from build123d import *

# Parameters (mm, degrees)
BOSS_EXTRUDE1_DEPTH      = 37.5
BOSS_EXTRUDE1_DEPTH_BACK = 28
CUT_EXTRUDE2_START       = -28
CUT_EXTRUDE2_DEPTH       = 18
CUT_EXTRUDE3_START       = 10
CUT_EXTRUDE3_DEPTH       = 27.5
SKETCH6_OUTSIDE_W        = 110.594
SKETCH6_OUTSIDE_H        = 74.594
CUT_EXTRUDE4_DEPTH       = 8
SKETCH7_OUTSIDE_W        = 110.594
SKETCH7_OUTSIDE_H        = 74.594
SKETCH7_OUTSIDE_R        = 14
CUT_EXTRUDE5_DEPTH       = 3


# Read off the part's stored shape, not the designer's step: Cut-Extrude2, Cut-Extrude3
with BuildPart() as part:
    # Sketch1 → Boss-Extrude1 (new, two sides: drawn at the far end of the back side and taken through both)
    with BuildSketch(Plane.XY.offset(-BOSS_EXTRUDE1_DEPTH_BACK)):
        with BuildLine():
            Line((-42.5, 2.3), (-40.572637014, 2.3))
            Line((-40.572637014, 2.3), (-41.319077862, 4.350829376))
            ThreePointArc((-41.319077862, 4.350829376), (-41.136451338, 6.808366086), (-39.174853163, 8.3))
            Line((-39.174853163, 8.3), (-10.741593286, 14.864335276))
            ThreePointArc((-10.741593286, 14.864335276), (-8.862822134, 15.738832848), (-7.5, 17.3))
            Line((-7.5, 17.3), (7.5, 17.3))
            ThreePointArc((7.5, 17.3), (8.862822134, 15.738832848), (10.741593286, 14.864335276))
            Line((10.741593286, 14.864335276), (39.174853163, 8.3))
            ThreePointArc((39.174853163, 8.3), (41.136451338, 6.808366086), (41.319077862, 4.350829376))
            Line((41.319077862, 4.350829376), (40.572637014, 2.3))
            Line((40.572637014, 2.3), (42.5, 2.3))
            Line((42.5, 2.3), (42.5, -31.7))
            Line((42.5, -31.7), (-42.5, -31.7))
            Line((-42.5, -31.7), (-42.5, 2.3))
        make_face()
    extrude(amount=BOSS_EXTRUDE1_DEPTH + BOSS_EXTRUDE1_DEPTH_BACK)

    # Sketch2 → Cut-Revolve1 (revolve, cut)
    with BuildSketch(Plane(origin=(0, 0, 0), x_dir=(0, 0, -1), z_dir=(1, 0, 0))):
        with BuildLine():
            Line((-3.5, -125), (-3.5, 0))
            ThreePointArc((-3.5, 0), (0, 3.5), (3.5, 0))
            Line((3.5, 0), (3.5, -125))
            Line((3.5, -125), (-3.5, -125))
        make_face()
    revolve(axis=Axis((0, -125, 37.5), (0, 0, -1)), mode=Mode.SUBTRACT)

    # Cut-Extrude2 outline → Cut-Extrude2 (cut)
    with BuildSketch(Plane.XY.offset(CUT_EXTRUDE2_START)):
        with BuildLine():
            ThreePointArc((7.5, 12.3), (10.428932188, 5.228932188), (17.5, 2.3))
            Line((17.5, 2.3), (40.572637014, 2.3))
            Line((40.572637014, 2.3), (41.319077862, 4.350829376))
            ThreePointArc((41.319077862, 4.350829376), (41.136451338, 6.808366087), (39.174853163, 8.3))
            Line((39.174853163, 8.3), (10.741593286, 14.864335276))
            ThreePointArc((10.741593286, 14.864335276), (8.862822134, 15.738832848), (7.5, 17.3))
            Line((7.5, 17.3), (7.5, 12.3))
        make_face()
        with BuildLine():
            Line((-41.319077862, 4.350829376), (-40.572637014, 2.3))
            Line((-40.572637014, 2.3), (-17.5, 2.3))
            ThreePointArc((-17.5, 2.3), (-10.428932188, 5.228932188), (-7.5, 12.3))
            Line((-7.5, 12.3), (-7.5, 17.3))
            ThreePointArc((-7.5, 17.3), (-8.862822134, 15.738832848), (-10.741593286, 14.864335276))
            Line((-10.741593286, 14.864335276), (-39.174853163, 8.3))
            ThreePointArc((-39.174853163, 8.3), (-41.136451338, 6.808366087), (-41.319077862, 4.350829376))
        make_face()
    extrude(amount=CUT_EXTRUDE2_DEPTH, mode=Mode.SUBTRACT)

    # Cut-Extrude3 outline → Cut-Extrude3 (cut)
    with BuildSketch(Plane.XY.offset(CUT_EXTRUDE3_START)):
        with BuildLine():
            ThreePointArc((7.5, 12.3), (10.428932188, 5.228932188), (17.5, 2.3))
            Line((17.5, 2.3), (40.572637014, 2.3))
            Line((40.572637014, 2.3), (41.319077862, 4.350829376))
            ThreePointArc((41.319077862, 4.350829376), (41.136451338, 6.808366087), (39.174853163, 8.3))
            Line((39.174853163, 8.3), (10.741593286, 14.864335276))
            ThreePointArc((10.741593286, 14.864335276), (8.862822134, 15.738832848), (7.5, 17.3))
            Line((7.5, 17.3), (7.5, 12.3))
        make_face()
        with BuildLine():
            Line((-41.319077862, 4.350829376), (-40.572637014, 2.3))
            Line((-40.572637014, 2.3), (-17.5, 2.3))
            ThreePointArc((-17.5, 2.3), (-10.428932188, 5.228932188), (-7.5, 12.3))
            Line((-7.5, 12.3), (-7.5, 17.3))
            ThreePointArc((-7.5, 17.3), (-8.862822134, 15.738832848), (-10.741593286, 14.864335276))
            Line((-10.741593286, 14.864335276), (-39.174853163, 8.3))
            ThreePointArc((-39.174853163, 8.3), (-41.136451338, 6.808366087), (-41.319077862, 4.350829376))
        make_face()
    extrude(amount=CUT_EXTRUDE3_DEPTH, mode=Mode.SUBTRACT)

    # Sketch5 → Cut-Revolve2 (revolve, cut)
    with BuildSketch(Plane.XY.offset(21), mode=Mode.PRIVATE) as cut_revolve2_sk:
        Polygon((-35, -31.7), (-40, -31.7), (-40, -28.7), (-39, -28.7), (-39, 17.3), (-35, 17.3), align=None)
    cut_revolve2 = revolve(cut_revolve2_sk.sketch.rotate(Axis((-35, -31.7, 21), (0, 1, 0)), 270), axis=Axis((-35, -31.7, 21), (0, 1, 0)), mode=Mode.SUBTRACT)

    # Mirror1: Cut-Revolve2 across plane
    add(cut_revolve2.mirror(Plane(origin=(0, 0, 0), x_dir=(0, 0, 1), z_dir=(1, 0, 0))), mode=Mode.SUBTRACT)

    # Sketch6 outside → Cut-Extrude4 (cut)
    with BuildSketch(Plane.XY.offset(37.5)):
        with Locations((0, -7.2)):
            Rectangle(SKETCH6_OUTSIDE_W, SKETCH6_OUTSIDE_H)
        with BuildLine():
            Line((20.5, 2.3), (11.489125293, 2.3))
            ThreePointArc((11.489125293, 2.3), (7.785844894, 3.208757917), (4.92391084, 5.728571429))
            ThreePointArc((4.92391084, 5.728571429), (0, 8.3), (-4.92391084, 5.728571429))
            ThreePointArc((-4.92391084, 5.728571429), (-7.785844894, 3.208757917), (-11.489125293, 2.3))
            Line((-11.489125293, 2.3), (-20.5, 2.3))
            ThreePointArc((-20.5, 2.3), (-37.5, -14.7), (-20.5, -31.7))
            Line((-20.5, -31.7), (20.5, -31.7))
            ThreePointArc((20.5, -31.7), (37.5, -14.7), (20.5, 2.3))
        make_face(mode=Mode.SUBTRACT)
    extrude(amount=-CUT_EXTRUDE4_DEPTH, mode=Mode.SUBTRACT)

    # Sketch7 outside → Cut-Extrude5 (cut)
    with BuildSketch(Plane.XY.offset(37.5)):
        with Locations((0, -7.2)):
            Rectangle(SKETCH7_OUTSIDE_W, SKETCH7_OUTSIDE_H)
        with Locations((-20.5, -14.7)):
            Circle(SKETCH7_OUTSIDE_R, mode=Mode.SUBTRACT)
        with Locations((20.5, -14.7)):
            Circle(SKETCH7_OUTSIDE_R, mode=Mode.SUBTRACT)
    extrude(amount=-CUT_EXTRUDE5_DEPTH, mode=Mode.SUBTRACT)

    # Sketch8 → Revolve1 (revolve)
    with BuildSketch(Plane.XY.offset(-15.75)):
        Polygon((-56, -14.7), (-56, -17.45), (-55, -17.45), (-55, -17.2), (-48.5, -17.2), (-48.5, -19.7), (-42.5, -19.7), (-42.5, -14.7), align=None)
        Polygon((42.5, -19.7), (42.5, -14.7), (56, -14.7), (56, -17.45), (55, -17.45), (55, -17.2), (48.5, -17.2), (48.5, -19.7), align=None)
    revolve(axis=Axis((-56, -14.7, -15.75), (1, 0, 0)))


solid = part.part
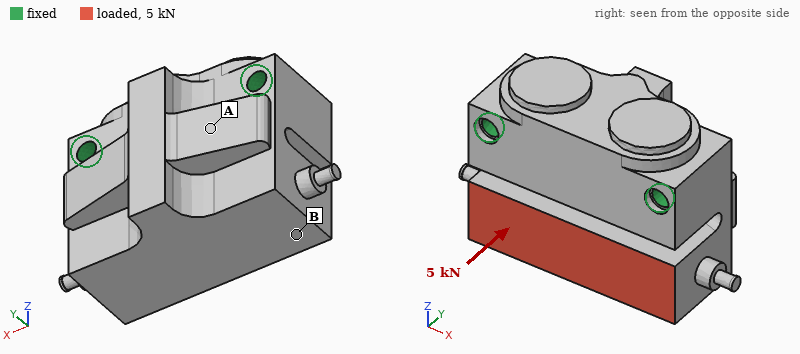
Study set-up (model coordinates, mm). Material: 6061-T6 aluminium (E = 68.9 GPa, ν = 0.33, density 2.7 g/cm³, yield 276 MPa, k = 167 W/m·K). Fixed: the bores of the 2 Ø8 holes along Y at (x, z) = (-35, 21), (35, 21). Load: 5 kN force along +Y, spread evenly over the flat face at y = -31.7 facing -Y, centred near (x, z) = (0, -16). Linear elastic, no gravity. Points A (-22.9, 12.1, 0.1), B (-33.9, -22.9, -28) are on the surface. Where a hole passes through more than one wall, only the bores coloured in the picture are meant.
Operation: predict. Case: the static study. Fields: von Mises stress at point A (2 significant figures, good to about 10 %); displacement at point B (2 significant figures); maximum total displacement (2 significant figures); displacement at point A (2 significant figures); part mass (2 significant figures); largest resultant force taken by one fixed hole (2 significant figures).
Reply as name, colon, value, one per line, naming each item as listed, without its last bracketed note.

von Mises stress at point A: 20 MPa
displacement at point B: 0.13 mm
maximum total displacement: 0.15 mm
displacement at point A: 0.036 mm
part mass: 510 g
largest resultant force taken by one fixed hole: 2.5 kN
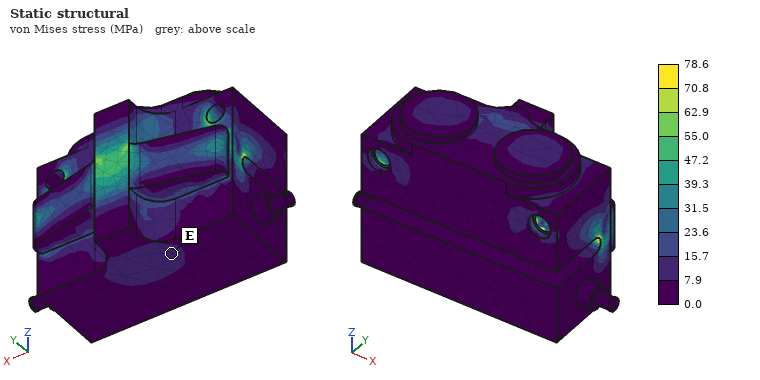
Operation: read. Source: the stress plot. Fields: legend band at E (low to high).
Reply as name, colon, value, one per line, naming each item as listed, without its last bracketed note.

legend band at E: 7.9 to 15.7 MPa
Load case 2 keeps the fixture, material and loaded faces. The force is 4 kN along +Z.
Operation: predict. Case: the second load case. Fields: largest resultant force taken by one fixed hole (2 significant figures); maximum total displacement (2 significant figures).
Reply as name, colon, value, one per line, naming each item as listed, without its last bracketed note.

largest resultant force taken by one fixed hole: 2.0 kN
maximum total displacement: 0.23 mm
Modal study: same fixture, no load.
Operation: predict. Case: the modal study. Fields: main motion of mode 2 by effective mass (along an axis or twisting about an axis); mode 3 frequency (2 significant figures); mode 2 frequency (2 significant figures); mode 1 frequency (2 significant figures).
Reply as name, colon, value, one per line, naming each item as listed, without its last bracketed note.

main motion of mode 2 by effective mass: along X
mode 3 frequency: 5900 Hz
mode 2 frequency: 4300 Hz
mode 1 frequency: 2100 Hz
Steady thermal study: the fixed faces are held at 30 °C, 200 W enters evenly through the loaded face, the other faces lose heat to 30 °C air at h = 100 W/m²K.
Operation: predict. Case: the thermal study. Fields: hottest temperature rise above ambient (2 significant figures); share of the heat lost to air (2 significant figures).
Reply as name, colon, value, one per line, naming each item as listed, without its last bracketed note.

hottest temperature rise above ambient: 51 K
share of the heat lost to air: 27 %
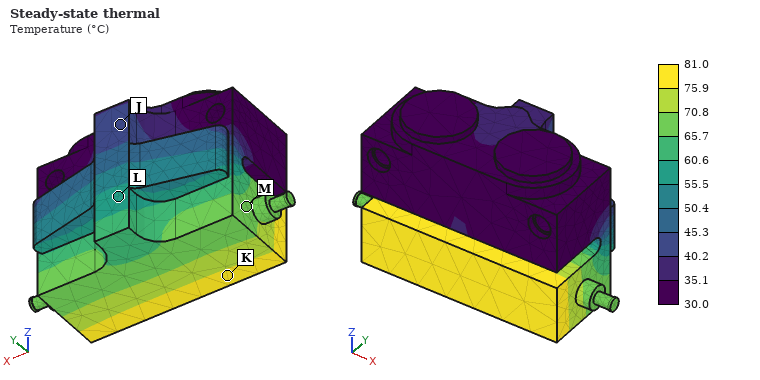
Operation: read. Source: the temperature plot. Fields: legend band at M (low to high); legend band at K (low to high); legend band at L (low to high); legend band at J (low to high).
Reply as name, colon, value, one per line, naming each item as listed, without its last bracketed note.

legend band at M: 65.7 to 70.8 °C
legend band at K: 75.9 to 81.0 °C
legend band at L: 55.5 to 60.6 °C
legend band at J: 40.2 to 45.3 °C
